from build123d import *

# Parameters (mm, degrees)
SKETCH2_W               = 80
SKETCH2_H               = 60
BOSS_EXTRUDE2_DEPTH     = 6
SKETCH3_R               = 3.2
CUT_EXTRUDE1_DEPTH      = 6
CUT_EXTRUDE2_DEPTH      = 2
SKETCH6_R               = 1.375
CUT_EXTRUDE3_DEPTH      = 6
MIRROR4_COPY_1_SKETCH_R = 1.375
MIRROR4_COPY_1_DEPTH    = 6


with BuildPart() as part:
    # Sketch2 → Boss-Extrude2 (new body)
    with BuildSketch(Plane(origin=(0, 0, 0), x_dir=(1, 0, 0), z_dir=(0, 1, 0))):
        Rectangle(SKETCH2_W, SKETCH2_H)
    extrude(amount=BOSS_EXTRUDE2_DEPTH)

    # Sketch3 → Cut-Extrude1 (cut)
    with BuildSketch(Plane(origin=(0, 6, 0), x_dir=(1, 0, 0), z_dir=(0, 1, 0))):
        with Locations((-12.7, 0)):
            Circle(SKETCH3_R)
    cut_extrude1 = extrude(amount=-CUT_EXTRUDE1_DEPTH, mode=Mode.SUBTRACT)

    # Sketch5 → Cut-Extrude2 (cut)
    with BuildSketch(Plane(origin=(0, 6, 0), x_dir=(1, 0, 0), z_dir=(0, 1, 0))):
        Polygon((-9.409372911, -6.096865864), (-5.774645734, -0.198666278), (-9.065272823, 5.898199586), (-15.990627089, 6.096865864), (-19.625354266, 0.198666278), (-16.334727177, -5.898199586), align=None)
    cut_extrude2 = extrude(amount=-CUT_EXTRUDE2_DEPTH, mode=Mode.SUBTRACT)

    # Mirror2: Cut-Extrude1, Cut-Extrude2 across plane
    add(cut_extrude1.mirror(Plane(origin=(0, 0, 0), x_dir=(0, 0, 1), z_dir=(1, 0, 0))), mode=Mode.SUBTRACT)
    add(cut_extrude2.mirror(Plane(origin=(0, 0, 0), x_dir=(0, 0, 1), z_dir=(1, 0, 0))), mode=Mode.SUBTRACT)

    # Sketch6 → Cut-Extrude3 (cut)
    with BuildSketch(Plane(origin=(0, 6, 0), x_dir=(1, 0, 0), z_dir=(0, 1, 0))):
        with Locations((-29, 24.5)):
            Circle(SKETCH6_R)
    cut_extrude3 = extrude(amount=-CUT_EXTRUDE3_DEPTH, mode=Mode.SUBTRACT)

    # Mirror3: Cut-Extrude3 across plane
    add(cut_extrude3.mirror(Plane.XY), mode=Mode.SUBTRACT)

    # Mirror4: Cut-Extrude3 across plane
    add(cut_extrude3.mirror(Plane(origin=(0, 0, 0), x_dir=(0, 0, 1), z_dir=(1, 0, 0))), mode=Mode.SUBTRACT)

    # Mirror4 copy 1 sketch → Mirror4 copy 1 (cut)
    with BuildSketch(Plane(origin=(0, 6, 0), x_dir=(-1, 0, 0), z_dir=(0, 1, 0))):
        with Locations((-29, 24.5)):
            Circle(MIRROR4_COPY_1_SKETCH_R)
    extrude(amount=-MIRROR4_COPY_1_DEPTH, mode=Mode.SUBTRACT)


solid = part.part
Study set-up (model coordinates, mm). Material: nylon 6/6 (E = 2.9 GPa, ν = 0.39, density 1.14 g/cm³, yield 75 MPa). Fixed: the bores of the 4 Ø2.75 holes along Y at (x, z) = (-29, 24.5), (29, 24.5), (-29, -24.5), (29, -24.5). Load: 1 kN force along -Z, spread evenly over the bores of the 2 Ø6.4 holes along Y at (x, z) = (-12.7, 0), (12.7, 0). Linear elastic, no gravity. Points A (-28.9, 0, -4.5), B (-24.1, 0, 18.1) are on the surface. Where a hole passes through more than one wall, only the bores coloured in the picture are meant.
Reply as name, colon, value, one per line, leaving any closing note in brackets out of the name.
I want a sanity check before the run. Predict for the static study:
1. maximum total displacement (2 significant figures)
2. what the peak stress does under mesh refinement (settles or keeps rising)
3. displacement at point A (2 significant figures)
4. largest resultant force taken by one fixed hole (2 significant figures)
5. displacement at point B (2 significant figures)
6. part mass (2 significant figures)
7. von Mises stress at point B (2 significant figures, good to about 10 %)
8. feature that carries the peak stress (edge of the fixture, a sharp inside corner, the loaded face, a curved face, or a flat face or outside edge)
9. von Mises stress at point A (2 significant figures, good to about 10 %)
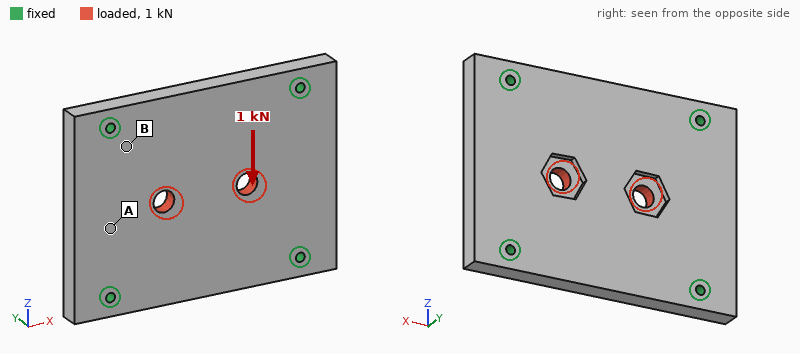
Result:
maximum total displacement: 51 µm
what the peak stress does under mesh refinement: keeps rising
displacement at point A: 14 µm
largest resultant force taken by one fixed hole: 280 N
displacement at point B: 13 µm
part mass: 32 g
von Mises stress at point B: 3.9 MPa
feature that carries the peak stress: edge of the fixture
von Mises stress at point A: 1.5 MPa
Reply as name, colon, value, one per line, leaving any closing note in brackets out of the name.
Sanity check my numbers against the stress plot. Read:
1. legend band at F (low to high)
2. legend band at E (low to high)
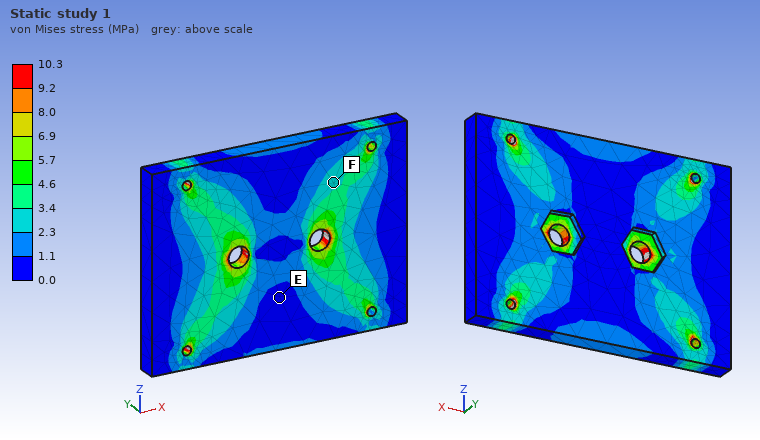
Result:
legend band at F: 2.3 to 3.4 MPa
legend band at E: 0.0 to 1.1 MPa
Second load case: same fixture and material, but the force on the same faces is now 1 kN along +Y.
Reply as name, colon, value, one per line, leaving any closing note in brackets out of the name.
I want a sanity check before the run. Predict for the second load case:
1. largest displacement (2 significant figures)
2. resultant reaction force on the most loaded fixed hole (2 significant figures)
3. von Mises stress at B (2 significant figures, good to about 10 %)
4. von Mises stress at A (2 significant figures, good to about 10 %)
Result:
largest displacement: 0.79 mm
resultant reaction force on the most loaded fixed hole: 260 N
von Mises stress at B: 9.6 MPa
von Mises stress at A: 11 MPa
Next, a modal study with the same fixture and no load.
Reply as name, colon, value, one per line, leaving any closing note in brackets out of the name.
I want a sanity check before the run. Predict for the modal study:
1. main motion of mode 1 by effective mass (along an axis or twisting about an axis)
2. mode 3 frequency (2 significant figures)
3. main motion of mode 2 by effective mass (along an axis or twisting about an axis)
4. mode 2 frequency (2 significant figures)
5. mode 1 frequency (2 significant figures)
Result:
main motion of mode 1 by effective mass: along Y
mode 3 frequency: 3200 Hz
main motion of mode 2 by effective mass: twisting about X
mode 2 frequency: 3000 Hz
mode 1 frequency: 2000 Hz
